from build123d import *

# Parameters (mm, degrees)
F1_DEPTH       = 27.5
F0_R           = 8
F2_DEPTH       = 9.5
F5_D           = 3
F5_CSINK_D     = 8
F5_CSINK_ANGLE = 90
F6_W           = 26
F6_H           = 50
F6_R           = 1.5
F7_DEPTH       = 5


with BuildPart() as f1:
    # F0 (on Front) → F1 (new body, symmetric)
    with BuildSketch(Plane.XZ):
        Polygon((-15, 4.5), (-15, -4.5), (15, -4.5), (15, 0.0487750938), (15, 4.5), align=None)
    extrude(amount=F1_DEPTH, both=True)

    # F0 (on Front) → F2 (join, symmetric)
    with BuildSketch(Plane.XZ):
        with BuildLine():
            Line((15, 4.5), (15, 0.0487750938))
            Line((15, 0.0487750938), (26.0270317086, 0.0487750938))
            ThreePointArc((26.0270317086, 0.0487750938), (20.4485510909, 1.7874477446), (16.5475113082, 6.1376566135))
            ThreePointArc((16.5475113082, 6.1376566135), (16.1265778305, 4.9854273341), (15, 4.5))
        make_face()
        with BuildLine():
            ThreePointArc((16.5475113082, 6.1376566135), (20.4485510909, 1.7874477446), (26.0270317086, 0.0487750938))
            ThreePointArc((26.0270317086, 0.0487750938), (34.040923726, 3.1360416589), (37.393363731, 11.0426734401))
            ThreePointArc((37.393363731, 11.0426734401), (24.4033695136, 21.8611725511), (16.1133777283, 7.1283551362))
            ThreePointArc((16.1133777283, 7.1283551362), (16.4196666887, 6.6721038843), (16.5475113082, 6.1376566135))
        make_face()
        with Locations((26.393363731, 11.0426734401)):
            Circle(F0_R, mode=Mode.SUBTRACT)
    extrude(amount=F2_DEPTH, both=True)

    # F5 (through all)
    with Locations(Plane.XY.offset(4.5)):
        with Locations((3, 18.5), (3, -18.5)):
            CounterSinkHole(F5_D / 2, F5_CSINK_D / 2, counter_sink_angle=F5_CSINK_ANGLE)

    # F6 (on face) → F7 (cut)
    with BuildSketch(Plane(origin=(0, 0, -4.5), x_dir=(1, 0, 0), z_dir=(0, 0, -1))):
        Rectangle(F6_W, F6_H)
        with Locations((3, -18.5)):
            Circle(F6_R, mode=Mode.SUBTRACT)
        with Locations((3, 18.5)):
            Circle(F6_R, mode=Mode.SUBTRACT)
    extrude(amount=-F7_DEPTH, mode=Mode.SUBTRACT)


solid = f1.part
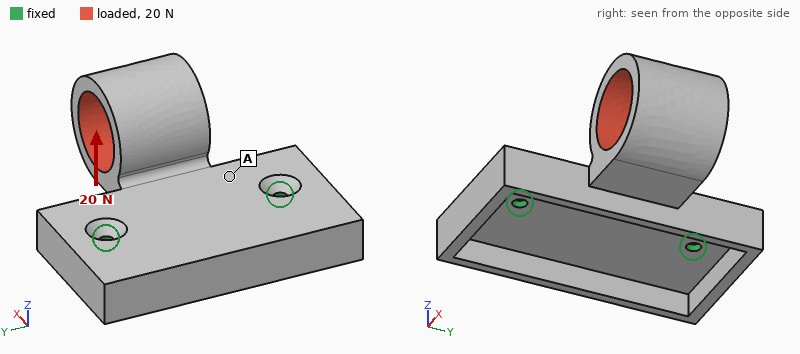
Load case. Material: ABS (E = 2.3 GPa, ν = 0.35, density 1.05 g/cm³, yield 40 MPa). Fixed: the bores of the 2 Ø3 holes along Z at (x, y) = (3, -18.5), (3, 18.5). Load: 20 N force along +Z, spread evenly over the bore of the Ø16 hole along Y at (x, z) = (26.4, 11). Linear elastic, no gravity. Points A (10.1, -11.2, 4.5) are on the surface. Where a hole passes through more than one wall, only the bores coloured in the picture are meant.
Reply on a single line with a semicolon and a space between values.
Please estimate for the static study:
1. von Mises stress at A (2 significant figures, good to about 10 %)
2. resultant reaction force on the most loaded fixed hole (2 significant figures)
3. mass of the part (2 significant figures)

2.6 MPa; 11 N; 13 g
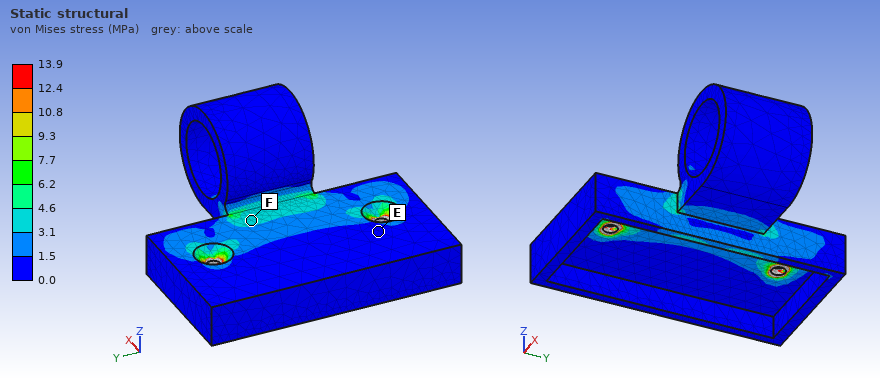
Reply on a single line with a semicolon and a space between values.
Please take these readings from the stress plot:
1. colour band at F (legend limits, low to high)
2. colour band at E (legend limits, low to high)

3.1 to 4.6 MPa; 0.0 to 1.5 MPa
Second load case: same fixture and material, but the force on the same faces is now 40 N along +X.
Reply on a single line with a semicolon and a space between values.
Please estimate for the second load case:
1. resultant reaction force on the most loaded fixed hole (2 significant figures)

20 N
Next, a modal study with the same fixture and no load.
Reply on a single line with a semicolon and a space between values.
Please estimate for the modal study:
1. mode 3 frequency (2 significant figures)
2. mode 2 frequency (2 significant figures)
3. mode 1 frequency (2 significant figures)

1600 Hz; 1400 Hz; 420 Hz
